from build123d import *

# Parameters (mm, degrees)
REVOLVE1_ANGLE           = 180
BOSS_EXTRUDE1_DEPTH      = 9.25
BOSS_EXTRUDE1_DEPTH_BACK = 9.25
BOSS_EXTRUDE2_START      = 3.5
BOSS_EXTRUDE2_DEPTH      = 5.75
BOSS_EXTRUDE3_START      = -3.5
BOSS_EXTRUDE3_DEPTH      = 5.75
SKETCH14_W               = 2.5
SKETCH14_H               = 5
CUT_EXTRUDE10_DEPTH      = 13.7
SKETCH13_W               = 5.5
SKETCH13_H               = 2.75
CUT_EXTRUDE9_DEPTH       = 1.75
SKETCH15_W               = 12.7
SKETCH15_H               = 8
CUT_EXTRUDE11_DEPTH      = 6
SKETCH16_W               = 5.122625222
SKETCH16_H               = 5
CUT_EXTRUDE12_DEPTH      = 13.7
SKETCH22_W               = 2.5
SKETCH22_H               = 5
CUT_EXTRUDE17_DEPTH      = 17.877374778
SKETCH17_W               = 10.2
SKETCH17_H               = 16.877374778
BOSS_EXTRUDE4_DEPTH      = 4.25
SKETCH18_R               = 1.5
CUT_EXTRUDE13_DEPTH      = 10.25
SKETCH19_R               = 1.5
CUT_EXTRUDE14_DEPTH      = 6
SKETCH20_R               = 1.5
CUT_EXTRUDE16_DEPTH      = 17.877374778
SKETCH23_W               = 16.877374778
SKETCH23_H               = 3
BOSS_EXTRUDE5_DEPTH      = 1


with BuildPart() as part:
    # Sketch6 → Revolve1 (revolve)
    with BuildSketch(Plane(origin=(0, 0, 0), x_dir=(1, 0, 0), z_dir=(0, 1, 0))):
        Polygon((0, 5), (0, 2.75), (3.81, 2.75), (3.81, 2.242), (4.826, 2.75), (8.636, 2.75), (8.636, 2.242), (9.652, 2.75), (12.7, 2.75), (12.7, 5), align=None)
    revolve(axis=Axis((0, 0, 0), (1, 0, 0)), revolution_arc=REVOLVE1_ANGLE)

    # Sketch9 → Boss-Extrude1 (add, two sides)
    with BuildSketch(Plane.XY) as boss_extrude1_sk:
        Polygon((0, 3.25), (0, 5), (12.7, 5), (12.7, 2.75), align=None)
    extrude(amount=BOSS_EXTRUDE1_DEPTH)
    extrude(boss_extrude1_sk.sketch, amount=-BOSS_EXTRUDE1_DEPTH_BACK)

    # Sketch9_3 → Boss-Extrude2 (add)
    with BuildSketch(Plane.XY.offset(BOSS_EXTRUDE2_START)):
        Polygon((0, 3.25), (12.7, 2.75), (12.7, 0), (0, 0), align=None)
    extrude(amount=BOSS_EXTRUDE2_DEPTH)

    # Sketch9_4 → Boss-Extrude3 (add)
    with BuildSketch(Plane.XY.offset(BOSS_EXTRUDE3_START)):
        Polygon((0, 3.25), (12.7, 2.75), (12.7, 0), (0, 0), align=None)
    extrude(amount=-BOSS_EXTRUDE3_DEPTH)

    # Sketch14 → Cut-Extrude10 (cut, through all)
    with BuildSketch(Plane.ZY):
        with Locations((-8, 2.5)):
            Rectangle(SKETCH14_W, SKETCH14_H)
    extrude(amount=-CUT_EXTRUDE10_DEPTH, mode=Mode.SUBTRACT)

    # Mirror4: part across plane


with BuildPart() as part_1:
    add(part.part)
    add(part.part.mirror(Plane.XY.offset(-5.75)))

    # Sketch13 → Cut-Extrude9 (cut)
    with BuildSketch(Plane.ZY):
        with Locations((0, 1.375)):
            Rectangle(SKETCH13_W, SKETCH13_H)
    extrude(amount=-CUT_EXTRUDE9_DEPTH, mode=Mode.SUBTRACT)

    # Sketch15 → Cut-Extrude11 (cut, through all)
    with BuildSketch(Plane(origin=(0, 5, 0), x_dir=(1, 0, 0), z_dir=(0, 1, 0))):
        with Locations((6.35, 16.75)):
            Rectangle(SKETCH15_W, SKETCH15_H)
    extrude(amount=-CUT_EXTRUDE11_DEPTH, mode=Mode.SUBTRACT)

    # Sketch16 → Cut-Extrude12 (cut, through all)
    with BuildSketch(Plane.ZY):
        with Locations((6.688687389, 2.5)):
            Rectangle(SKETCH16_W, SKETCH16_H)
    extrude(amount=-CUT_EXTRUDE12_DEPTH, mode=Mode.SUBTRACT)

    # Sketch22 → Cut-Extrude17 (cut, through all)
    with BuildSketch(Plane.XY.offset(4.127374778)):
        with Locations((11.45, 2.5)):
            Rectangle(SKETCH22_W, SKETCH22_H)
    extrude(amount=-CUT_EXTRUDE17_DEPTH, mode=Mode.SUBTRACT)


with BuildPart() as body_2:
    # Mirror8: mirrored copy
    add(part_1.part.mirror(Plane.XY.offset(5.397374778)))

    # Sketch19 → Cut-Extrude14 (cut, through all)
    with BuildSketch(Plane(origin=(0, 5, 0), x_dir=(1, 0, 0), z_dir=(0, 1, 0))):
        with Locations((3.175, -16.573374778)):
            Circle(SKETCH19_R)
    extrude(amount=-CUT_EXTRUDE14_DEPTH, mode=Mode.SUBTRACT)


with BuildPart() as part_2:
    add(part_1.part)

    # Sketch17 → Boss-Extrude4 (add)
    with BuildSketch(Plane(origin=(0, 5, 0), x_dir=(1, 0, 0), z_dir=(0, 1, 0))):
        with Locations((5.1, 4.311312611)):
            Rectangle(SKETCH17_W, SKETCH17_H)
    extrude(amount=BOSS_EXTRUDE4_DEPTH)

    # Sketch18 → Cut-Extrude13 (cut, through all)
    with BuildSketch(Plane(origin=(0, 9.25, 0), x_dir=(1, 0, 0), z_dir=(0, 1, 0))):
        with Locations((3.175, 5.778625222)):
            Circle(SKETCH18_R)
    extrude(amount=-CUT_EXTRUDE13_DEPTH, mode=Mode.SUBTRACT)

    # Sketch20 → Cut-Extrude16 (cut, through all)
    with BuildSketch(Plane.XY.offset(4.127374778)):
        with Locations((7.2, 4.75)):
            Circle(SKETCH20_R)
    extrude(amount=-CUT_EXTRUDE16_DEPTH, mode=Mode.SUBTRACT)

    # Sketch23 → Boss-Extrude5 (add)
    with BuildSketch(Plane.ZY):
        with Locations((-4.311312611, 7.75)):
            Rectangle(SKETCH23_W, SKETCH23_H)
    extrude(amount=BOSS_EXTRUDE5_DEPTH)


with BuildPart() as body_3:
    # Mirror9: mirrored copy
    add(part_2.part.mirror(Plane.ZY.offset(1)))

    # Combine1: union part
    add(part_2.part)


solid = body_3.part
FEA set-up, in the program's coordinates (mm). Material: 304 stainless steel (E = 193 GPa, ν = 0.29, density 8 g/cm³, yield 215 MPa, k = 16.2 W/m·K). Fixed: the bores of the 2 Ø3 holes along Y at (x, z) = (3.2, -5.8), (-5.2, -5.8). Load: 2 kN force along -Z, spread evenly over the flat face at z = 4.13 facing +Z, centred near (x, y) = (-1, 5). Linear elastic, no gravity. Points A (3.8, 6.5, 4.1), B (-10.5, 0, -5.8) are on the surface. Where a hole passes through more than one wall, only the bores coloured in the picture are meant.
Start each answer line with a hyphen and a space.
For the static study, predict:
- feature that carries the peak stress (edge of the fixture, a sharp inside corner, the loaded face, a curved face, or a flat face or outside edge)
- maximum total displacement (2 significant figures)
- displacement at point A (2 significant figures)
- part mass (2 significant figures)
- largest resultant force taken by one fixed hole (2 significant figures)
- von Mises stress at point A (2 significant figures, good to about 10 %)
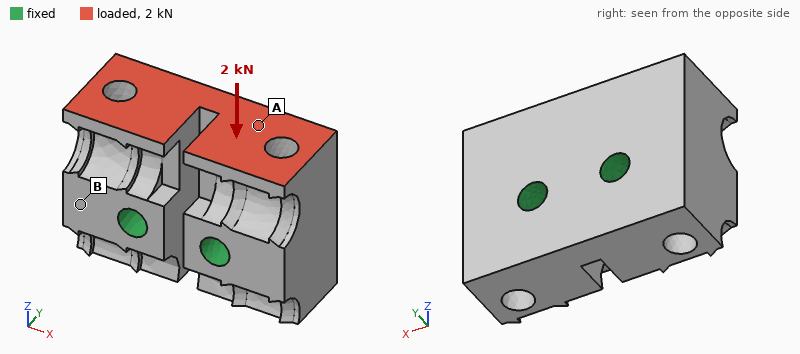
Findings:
- a sharp inside corner
- 4.3 µm
- 1.0 µm
- 20 g
- 1.0 kN
- 20 MPa
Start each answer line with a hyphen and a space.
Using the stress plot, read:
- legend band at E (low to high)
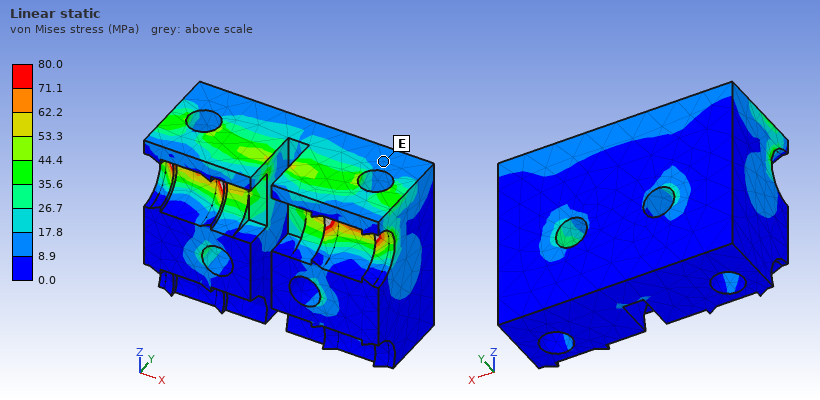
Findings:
- 8.9 to 17.8 MPa
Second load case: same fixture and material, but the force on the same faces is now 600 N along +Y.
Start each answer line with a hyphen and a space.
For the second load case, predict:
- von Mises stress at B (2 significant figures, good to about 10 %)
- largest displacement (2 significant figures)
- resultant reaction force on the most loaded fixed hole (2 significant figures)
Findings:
- 5.3 MPa
- 3.1 µm
- 300 N
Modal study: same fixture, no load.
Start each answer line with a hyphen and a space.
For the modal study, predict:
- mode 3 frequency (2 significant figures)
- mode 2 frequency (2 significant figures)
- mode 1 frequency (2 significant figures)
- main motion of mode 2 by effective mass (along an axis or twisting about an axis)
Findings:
- 48 kHz
- 43 kHz
- 40 kHz
- along Y
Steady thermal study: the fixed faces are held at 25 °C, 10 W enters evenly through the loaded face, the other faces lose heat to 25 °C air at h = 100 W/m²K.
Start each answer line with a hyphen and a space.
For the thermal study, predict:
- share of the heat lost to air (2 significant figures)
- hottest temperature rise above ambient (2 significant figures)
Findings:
- 20 %
- 47 K
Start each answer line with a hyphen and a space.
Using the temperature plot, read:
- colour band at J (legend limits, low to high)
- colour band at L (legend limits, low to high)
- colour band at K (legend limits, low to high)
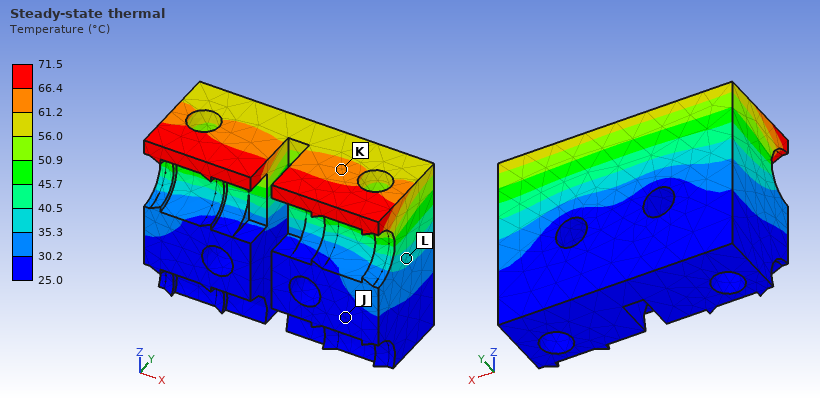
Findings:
- 25.0 to 30.2 °C
- 35.3 to 40.5 °C
- 61.2 to 66.4 °C
